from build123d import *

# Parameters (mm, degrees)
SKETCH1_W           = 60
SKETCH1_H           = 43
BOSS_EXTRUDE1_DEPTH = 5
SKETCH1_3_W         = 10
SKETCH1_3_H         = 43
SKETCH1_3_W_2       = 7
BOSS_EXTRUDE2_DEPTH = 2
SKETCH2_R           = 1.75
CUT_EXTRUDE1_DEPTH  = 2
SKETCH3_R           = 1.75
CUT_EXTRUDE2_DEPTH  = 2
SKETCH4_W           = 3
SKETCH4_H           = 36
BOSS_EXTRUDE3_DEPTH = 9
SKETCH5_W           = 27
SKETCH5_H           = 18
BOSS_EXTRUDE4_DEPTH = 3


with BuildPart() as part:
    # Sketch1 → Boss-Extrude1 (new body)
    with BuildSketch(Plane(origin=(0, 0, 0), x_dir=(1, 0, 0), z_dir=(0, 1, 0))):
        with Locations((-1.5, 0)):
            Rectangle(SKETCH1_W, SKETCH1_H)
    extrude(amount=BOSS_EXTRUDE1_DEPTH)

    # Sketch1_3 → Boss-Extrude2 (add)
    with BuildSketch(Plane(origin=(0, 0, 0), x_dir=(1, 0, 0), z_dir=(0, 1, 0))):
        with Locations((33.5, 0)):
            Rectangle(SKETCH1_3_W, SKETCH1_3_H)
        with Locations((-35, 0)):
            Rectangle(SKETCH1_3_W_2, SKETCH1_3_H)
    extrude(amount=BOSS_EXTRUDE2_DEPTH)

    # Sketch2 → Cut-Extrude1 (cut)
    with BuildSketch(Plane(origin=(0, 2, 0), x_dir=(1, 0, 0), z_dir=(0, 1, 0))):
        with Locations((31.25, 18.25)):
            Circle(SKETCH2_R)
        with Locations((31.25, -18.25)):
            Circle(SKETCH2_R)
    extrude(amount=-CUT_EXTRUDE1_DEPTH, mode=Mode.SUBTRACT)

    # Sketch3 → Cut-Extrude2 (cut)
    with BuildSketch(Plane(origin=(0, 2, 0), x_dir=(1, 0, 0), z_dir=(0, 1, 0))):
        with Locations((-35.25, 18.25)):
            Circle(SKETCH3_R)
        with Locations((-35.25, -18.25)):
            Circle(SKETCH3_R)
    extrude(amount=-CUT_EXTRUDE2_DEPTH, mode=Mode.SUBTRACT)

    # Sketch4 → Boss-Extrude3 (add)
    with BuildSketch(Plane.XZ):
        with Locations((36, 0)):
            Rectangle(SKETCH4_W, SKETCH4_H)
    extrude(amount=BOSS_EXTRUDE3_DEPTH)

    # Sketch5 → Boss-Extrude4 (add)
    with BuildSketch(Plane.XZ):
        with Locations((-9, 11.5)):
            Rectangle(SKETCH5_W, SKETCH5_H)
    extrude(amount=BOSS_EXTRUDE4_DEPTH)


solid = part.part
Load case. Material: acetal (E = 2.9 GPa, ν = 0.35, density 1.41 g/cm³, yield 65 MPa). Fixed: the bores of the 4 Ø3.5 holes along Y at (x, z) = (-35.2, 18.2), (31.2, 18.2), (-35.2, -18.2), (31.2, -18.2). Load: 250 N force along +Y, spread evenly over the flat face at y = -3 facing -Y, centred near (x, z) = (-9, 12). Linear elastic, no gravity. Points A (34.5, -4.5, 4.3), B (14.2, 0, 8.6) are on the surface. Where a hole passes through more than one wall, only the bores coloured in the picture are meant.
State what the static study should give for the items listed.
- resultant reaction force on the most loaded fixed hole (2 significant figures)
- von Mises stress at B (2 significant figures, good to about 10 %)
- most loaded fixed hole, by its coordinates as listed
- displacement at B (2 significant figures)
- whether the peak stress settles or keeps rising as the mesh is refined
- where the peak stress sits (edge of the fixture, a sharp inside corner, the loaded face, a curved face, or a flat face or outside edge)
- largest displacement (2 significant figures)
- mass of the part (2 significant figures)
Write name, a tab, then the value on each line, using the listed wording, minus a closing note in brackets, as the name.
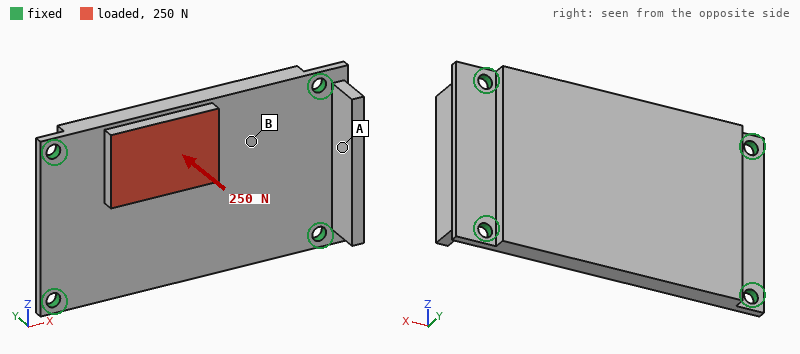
resultant reaction force on the most loaded fixed hole	170 N
von Mises stress at B	5.6 MPa
most loaded fixed hole, by its coordinates as listed	(-35.2, 18.2)
displacement at B	0.33 mm
whether the peak stress settles or keeps rising as the mesh is refined	keeps rising
where the peak stress sits	edge of the fixture
largest displacement	0.58 mm
mass of the part	24 g
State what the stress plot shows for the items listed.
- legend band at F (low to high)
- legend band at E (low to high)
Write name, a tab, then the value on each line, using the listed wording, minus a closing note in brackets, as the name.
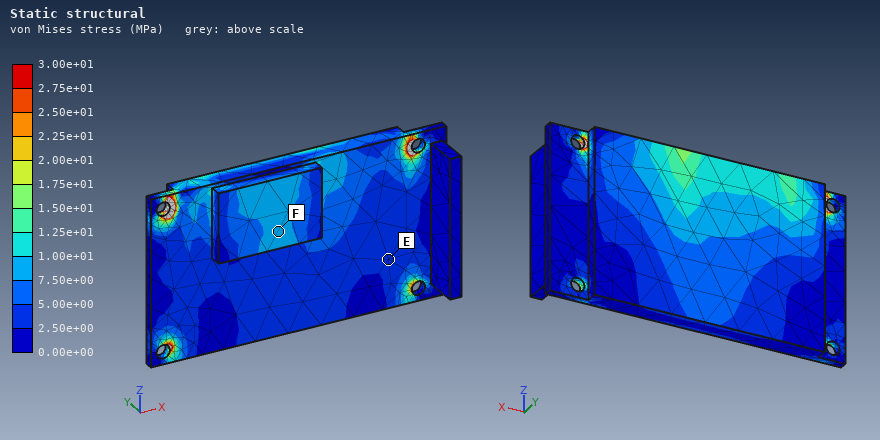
legend band at F	7.50e+00 to 1.00e+01 MPa
legend band at E	2.50e+00 to 5.00e+00 MPa
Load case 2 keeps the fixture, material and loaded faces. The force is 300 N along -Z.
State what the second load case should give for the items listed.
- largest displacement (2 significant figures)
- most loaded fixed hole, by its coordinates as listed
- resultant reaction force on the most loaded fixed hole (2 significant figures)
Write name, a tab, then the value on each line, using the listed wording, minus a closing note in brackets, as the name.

largest displacement	0.18 mm
most loaded fixed hole, by its coordinates as listed	(-35.2, 18.2)
resultant reaction force on the most loaded fixed hole	110 N
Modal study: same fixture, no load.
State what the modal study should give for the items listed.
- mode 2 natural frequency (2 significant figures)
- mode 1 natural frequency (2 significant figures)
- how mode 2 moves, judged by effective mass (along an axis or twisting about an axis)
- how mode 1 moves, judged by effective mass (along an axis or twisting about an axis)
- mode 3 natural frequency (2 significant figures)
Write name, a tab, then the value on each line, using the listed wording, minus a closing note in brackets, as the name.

mode 2 natural frequency	1800 Hz
mode 1 natural frequency	1100 Hz
how mode 2 moves, judged by effective mass	twisting about X
how mode 1 moves, judged by effective mass	along Y
mode 3 natural frequency	2600 Hz
